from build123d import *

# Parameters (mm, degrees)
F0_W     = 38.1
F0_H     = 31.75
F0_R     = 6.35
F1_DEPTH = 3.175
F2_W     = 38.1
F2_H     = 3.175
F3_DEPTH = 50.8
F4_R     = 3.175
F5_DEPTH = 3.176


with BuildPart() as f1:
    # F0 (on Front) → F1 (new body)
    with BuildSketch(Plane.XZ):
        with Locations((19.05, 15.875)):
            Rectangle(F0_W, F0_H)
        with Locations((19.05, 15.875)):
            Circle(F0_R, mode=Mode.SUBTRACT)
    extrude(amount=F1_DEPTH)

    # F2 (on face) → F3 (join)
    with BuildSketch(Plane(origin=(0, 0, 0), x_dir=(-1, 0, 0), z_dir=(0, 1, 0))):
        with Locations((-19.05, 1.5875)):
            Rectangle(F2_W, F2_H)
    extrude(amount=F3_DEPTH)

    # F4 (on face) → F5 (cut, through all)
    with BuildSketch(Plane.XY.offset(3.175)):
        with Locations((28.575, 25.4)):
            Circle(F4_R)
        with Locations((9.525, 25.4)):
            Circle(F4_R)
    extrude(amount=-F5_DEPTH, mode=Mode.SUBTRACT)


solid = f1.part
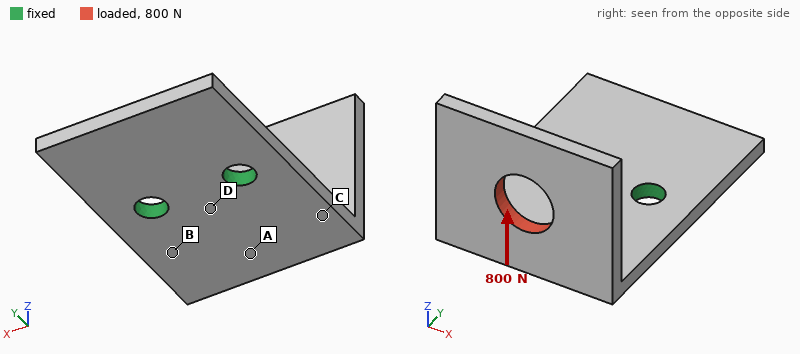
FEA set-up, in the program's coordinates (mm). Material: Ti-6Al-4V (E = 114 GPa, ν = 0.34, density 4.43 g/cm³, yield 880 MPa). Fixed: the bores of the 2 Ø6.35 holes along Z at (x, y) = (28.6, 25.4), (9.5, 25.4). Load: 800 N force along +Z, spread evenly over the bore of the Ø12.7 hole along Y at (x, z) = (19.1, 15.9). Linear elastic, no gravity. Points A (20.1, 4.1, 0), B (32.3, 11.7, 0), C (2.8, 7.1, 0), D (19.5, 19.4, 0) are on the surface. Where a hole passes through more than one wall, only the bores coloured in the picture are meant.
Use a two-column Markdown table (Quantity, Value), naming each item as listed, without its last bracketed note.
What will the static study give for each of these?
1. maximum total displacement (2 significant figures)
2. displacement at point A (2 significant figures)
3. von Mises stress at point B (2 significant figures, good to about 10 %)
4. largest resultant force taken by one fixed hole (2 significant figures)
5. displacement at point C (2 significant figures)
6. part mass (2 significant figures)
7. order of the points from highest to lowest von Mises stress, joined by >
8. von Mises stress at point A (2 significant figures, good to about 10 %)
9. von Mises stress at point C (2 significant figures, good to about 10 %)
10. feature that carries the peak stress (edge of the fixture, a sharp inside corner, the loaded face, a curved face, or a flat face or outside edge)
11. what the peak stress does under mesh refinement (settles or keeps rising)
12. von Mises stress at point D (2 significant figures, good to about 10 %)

| Quantity | Value |
|---|---|
| maximum total displacement | 0.73 mm |
| displacement at point A | 0.24 mm |
| von Mises stress at point B | 150 MPa |
| largest resultant force taken by one fixed hole | 400 N |
| displacement at point C | 0.18 mm |
| part mass | 42 g |
| order of the points from highest to lowest von Mises stress, joined by > | D > B > C > A |
| von Mises stress at point A | 65 MPa |
| von Mises stress at point C | 110 MPa |
| feature that carries the peak stress | edge of the fixture |
| what the peak stress does under mesh refinement | keeps rising |
| von Mises stress at point D | 200 MPa |
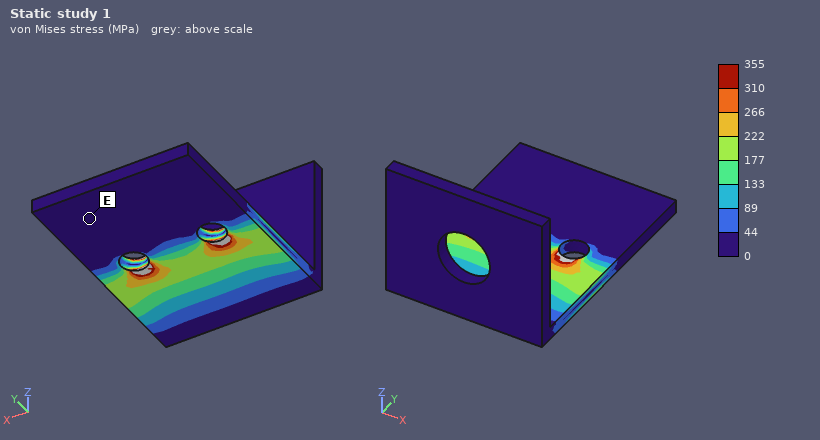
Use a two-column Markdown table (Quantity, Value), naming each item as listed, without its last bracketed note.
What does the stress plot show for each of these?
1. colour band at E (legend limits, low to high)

| Quantity | Value |
|---|---|
| colour band at E | 0 to 44 MPa |
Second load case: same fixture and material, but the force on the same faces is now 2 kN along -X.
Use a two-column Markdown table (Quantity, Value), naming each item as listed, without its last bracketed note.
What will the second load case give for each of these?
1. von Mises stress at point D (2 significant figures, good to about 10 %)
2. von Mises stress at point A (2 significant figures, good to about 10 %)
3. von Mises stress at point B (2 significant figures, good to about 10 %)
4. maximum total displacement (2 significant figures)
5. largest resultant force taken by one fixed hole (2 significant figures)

| Quantity | Value |
|---|---|
| von Mises stress at point D | 93 MPa |
| von Mises stress at point A | 200 MPa |
| von Mises stress at point B | 220 MPa |
| maximum total displacement | 0.85 mm |
| largest resultant force taken by one fixed hole | 2.7 kN |
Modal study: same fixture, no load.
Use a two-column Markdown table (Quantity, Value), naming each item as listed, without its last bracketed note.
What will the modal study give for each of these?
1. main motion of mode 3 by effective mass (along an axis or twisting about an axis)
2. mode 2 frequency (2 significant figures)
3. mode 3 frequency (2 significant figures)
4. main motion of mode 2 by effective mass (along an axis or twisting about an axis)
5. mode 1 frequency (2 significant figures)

| Quantity | Value |
|---|---|
| main motion of mode 3 by effective mass | along Z |
| mode 2 frequency | 2100 Hz |
| mode 3 frequency | 3200 Hz |
| main motion of mode 2 by effective mass | along X |
| mode 1 frequency | 1200 Hz |
